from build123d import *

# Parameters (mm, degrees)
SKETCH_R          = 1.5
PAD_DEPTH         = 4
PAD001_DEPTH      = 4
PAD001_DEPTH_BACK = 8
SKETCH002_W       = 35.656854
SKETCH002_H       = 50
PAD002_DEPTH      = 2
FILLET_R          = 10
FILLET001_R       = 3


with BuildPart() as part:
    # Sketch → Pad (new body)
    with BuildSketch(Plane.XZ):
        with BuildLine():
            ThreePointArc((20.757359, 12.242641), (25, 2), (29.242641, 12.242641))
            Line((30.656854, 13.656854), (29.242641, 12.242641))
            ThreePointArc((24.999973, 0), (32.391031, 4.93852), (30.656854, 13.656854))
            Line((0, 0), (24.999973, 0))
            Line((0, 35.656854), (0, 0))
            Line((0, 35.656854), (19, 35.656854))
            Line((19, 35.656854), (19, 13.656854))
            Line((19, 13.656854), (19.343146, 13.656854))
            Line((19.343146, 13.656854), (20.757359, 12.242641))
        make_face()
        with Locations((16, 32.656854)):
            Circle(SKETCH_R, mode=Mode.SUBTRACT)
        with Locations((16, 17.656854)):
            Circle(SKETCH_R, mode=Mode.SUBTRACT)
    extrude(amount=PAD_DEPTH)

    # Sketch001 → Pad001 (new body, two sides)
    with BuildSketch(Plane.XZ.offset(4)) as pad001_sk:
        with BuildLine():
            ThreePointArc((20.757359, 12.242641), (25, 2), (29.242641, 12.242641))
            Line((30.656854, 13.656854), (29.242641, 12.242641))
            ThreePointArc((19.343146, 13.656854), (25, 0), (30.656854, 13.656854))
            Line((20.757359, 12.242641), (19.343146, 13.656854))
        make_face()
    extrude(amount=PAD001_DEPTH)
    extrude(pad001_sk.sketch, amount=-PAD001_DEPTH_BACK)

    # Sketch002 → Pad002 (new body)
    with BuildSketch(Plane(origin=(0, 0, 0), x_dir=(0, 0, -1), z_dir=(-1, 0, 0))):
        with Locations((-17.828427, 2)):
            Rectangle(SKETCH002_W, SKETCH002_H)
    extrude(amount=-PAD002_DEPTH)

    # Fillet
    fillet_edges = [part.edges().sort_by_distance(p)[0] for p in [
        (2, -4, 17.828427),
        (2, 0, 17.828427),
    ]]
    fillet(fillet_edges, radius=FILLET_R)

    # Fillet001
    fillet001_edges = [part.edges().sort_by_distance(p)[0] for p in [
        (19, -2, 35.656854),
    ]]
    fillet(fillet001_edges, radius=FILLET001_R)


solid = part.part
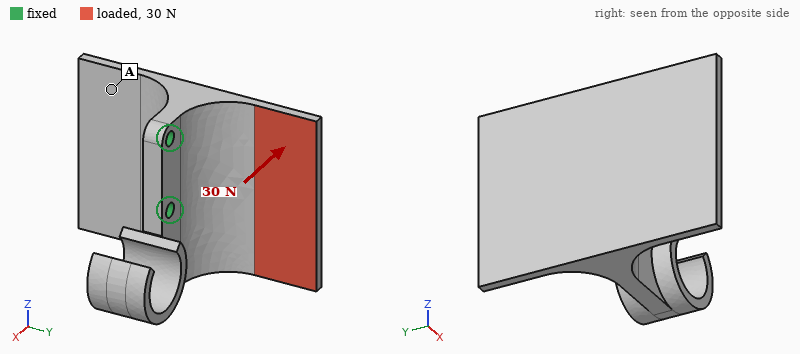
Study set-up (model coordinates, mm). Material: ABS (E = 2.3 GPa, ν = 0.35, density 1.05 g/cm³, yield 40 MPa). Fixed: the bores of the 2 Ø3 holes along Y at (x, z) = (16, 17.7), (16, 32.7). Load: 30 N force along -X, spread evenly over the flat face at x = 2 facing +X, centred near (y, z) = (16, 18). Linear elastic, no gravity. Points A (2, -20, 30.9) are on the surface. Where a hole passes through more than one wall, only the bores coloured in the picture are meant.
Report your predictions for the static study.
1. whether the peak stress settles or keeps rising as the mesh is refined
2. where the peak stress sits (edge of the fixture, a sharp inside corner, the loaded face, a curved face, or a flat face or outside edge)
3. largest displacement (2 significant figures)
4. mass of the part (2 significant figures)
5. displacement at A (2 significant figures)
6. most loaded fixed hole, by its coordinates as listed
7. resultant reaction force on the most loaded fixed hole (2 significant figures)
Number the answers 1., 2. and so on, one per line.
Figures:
1. keeps rising
2. edge of the fixture
3. 0.78 mm
4. 8.6 g
5. 0.25 mm
6. (16, 17.7)
7. 28 N
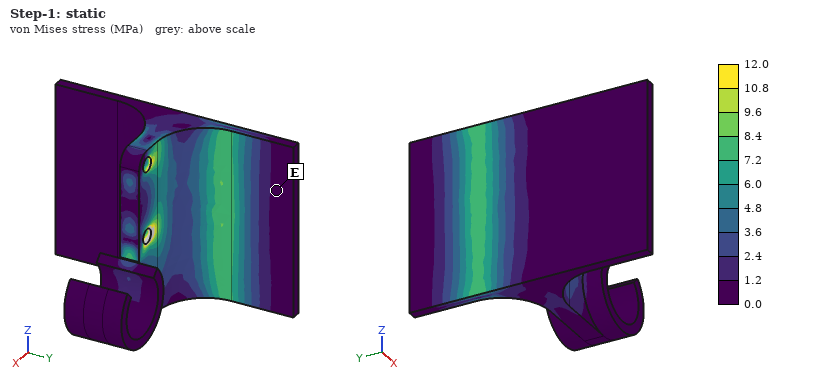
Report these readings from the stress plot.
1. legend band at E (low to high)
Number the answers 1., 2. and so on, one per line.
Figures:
1. 0.0 to 1.2 MPa
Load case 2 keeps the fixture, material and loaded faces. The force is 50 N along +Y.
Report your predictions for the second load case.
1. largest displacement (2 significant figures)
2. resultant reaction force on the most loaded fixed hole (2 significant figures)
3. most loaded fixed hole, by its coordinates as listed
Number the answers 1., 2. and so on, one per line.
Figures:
1. 0.39 mm
2. 45 N
3. (16, 17.7)
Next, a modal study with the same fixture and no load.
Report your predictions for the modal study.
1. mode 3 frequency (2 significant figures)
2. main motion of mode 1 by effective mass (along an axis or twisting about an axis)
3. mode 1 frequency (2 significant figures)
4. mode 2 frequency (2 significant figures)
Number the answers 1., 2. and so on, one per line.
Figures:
1. 1300 Hz
2. along Y
3. 770 Hz
4. 1300 Hz
